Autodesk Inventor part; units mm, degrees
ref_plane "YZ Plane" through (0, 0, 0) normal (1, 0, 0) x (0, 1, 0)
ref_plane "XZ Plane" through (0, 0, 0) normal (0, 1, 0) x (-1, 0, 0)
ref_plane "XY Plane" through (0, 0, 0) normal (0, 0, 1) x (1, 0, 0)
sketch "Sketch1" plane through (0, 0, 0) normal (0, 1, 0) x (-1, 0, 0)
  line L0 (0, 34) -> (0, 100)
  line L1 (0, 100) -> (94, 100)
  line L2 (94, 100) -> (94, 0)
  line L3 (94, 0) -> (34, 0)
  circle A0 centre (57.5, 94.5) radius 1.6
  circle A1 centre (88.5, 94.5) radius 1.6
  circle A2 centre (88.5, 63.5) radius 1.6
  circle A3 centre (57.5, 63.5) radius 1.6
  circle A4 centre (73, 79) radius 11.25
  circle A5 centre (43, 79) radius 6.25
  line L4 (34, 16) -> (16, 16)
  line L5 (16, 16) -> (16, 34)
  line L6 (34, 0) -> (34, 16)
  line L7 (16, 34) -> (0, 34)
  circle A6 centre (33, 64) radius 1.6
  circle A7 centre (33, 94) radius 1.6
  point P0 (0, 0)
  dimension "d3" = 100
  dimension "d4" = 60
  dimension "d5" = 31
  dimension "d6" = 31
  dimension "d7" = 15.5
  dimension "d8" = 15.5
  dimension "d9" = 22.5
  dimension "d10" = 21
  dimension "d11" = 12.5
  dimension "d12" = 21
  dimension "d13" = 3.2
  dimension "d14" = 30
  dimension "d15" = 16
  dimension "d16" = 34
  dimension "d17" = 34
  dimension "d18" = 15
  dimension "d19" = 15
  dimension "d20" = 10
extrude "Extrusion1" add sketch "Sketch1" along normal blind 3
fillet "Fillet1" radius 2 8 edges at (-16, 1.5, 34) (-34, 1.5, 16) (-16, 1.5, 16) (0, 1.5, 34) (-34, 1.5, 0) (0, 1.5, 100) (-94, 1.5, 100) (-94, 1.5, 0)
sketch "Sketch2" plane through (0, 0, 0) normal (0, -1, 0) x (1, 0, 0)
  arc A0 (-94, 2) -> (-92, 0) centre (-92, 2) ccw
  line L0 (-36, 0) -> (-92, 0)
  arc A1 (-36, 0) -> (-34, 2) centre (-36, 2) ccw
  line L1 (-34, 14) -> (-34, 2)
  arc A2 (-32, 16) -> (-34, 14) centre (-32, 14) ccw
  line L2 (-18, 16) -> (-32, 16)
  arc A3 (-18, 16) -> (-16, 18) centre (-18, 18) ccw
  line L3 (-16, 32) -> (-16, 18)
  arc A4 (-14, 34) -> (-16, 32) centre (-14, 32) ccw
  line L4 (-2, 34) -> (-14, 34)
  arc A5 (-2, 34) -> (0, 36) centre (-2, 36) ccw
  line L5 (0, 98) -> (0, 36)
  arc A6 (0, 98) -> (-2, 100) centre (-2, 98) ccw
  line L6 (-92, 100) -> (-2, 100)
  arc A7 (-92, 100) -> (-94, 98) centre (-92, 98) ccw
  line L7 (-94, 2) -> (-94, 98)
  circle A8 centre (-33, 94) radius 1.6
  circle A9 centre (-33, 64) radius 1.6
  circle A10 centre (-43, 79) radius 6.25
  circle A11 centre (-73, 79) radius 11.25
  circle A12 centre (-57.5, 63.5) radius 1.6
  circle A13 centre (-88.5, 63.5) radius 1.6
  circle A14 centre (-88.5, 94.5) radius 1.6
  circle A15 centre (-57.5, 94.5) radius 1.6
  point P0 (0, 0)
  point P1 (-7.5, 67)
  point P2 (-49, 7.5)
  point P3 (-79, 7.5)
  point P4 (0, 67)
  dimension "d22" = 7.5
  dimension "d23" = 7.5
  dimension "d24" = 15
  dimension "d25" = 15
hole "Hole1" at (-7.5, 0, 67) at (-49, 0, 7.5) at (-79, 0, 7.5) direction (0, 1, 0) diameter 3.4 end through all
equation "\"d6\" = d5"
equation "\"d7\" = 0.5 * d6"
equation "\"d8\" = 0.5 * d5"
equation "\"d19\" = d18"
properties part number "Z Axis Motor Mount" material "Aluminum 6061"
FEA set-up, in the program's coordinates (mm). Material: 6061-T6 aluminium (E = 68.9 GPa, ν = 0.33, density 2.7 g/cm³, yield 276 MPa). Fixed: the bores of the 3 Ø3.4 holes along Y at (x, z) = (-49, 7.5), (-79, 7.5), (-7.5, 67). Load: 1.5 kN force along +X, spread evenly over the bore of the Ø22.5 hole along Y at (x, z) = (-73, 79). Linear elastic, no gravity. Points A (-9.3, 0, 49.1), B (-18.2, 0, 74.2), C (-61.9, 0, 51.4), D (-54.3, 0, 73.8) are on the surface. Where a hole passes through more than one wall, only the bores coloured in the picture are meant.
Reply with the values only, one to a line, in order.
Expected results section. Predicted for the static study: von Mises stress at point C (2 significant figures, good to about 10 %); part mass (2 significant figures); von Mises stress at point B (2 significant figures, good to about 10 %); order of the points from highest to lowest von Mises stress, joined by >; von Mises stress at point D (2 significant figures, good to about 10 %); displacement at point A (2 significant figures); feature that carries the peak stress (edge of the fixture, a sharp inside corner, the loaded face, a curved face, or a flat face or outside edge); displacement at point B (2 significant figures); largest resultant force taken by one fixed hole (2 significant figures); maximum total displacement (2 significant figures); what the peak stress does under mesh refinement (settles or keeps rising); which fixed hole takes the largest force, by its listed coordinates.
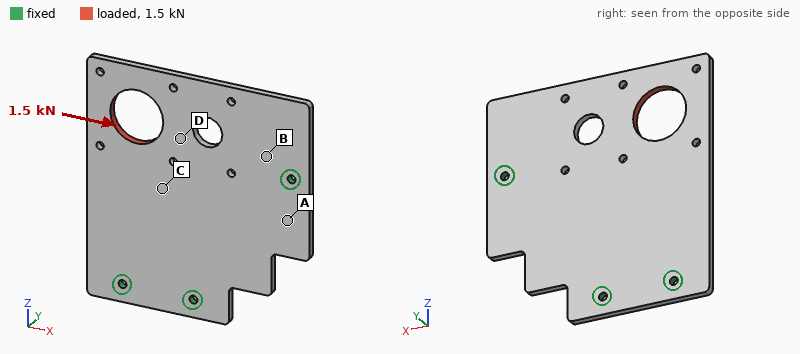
7.7 MPa
65 g
17 MPa
B > D > C > A
13 MPa
4.3 µm
edge of the fixture
5.5 µm
1.3 kN
26 µm
keeps rising
(-7.5, 67)
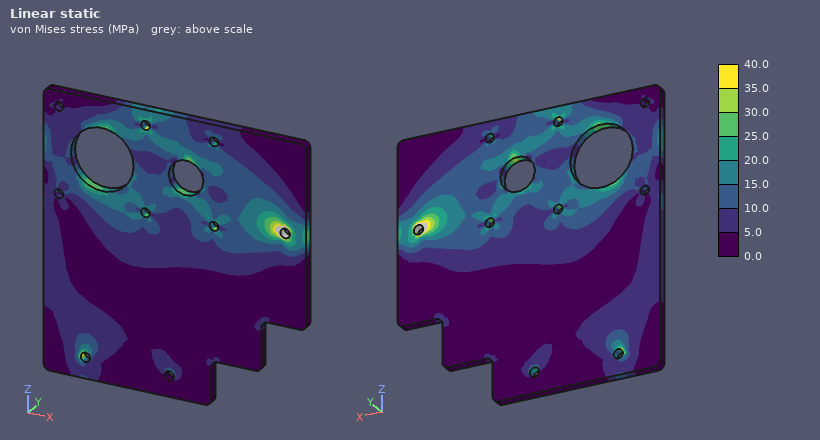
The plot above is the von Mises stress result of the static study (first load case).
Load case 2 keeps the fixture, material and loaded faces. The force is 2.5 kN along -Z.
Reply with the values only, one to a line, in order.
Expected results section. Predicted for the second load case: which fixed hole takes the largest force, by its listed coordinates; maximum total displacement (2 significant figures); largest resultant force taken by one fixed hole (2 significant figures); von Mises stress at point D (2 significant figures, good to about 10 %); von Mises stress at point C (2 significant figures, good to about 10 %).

(-79, 7.5)
36 µm
1.4 kN
18 MPa
15 MPa
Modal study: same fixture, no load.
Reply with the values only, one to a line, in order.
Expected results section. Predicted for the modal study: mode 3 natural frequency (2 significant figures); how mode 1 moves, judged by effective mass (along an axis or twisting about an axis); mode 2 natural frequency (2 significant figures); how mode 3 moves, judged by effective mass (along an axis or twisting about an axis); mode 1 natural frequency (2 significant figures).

2000 Hz
along Y
1600 Hz
along Y
570 Hz
